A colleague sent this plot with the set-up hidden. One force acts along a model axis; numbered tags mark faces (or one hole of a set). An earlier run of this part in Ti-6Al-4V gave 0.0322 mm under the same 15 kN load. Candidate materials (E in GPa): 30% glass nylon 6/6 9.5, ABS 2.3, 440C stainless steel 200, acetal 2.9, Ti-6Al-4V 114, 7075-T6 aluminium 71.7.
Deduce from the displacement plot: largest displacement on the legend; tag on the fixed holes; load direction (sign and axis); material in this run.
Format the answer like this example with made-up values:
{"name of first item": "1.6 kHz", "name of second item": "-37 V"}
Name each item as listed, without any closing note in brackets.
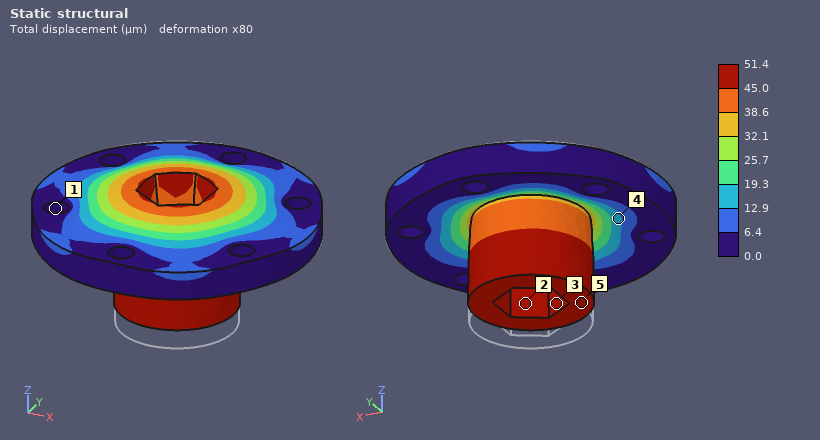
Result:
{"largest displacement on the legend": "51.4 µm", "tag on the fixed holes": "1", "load direction": "+Z", "material in this run": "7075-T6 aluminium"}
